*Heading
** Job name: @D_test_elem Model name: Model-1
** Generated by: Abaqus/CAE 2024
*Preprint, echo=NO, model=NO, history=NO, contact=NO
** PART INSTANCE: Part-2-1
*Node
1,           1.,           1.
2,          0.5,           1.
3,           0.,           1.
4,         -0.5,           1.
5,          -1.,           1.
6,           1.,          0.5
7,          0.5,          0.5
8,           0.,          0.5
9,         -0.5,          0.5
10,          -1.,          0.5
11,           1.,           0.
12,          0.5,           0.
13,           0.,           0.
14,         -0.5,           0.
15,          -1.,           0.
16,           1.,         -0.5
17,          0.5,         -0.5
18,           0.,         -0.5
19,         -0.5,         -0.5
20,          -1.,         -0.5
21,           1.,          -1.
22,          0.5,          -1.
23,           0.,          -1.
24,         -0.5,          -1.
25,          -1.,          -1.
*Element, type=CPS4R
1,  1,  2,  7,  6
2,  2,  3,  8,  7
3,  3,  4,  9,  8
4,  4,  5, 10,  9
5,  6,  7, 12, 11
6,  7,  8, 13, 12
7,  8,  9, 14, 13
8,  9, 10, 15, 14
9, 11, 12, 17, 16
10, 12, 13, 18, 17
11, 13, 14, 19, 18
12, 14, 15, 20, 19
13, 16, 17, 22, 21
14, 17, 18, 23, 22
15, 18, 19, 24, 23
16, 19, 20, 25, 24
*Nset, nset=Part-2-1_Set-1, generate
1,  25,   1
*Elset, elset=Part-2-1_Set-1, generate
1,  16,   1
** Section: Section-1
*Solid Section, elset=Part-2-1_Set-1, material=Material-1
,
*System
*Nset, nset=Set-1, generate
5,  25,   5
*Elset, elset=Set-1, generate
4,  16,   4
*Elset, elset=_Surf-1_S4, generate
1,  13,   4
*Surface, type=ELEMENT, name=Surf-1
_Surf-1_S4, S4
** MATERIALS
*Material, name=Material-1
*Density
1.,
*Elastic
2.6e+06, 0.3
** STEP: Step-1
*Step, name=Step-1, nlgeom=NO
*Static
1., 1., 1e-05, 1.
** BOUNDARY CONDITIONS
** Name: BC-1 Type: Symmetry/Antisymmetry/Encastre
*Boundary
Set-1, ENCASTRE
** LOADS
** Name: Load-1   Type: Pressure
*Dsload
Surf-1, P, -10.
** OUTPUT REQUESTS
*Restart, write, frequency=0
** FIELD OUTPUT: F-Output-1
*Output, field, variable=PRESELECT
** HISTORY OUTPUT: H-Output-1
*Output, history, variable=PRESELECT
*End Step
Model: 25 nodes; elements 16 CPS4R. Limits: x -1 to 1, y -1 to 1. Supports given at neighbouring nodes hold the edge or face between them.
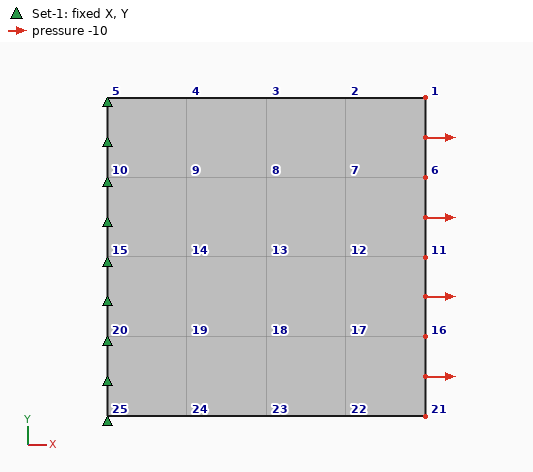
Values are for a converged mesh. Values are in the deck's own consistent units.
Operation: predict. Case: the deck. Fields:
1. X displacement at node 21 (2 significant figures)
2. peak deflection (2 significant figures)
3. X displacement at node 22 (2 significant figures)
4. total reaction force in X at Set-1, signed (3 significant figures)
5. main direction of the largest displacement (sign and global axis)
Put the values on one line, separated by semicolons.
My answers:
7.6e-06; 7.7e-06; 5.7e-06; -20.0; +X
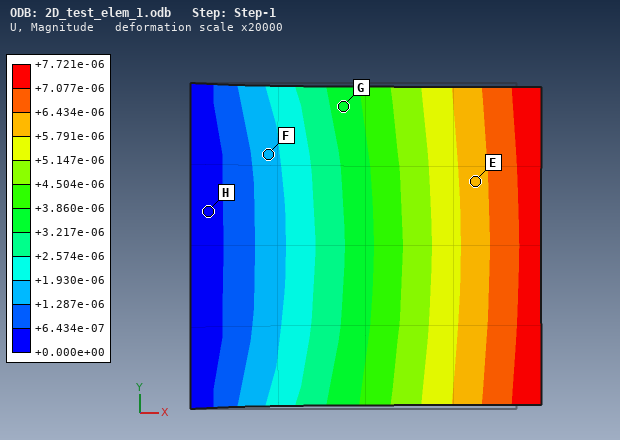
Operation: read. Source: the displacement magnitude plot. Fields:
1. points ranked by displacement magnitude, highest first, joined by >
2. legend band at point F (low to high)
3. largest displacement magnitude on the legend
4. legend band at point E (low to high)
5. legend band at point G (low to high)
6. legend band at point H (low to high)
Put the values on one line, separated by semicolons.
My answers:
E > G > F > H; +1.287e-06 to +1.930e-06; +7.721e-06; +5.791e-06 to +6.434e-06; +3.217e-06 to +3.860e-06; +0.000e+00 to +6.434e-07
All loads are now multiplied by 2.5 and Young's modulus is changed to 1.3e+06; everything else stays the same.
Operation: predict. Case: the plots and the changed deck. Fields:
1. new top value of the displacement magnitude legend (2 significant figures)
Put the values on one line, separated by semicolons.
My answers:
3.9e-05
